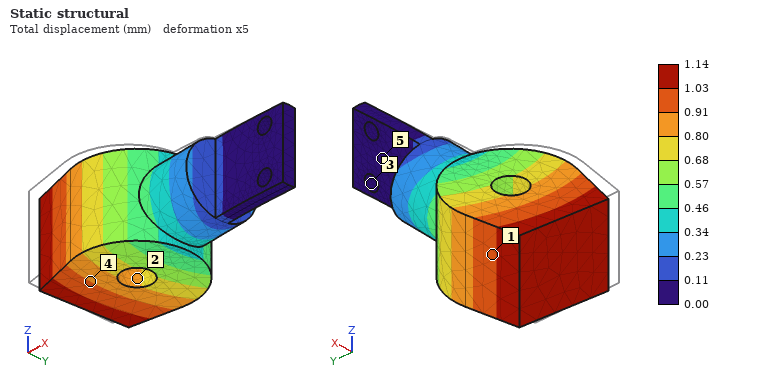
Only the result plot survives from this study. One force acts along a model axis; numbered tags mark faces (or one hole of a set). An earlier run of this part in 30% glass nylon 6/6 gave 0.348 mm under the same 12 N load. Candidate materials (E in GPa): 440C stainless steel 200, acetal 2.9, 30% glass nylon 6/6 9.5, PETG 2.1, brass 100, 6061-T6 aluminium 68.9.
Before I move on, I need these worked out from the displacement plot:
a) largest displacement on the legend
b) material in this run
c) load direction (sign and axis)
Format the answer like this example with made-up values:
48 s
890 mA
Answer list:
1.14 mm
acetal
+Y
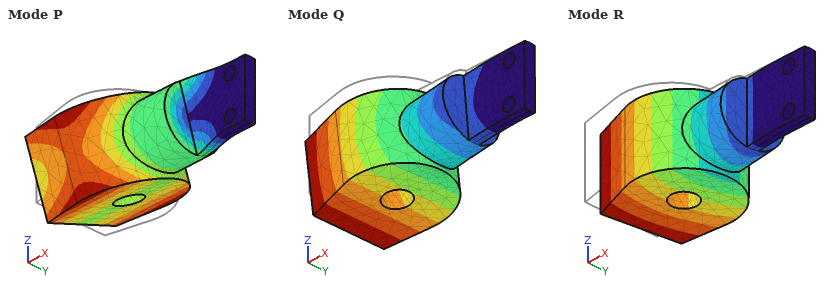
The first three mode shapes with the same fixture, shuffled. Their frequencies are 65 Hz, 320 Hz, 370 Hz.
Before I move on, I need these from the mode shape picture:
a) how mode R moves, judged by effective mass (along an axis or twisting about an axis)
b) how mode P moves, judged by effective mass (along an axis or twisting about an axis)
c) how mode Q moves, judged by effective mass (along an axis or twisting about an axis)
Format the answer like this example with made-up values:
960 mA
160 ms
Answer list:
along Y
twisting about X
along Z
